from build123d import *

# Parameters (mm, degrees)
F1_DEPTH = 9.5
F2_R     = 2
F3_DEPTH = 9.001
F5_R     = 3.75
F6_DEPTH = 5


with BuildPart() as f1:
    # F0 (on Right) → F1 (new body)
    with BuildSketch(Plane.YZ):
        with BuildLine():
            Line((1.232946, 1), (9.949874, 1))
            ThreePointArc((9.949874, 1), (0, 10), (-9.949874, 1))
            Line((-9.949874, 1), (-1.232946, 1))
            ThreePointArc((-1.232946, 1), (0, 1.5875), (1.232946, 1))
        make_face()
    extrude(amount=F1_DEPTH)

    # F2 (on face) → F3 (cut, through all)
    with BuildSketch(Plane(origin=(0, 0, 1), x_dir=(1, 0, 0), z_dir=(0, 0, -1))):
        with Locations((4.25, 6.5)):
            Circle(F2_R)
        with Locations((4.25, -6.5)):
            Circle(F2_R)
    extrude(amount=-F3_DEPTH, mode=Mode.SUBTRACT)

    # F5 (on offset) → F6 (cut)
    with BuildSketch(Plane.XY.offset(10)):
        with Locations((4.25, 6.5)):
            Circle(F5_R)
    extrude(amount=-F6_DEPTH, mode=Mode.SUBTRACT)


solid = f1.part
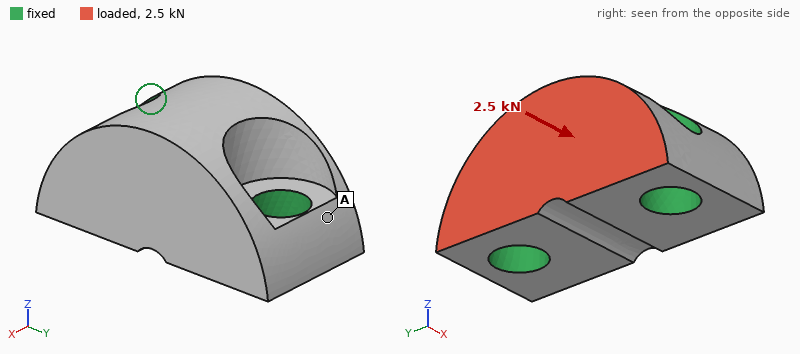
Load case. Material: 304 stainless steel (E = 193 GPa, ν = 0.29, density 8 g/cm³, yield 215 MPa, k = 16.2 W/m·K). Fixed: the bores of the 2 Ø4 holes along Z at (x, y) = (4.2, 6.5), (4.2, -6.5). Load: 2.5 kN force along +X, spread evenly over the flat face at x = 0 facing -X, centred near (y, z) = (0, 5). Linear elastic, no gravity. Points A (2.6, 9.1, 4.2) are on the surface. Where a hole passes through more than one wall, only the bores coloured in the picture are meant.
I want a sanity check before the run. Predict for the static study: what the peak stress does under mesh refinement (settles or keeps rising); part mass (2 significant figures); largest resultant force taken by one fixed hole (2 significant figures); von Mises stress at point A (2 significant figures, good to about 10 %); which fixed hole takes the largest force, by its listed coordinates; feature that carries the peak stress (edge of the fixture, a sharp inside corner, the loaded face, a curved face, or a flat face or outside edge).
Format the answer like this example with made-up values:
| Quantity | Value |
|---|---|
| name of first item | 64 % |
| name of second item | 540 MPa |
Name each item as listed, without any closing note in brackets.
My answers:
| Quantity | Value |
|---|---|
| what the peak stress does under mesh refinement | keeps rising |
| part mass | 8.5 g |
| largest resultant force taken by one fixed hole | 1.4 kN |
| von Mises stress at point A | 28 MPa |
| which fixed hole takes the largest force, by its listed coordinates | (4.2, -6.5) |
| feature that carries the peak stress | a sharp inside corner |
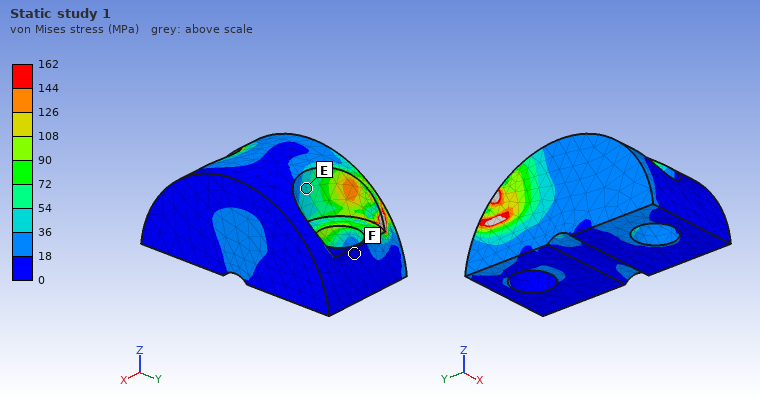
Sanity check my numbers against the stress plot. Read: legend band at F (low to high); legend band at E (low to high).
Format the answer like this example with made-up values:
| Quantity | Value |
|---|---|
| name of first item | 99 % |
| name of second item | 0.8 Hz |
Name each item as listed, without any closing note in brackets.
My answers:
| Quantity | Value |
|---|---|
| legend band at F | 0 to 18 MPa |
| legend band at E | 36 to 54 MPa |
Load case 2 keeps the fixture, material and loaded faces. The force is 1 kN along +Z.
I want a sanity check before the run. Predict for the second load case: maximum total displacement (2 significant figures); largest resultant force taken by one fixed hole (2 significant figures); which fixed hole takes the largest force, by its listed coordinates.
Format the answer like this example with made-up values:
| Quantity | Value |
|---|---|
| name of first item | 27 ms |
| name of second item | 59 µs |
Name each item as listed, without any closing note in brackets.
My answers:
| Quantity | Value |
|---|---|
| maximum total displacement | 2.4 µm |
| largest resultant force taken by one fixed hole | 550 N |
| which fixed hole takes the largest force, by its listed coordinates | (4.2, -6.5) |
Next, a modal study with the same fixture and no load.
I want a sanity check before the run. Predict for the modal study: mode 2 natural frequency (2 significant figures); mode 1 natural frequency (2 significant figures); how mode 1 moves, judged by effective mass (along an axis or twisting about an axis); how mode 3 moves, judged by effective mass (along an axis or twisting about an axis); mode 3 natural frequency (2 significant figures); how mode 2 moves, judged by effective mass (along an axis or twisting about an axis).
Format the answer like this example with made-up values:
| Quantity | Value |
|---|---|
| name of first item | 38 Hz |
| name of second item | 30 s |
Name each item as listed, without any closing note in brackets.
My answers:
| Quantity | Value |
|---|---|
| mode 2 natural frequency | 91 kHz |
| mode 1 natural frequency | 69 kHz |
| how mode 1 moves, judged by effective mass | along X |
| how mode 3 moves, judged by effective mass | along X |
| mode 3 natural frequency | 110 kHz |
| how mode 2 moves, judged by effective mass | along Z |
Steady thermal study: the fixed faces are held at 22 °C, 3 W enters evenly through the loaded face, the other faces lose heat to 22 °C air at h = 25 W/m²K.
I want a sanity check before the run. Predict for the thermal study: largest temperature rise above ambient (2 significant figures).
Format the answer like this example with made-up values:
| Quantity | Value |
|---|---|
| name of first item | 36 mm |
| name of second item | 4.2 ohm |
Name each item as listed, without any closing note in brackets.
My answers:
| Quantity | Value |
|---|---|
| largest temperature rise above ambient | 13 K |
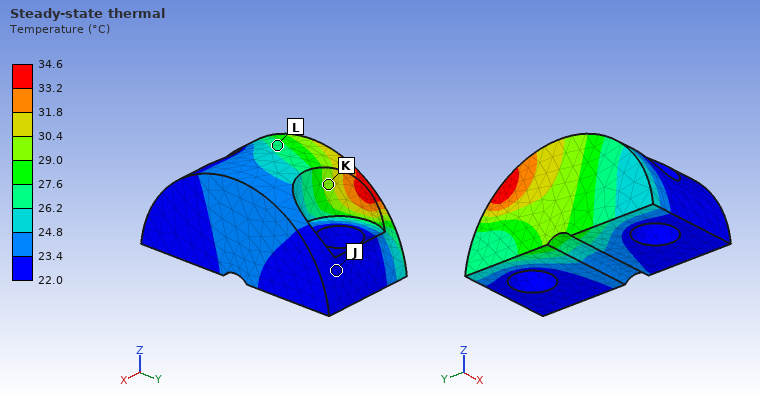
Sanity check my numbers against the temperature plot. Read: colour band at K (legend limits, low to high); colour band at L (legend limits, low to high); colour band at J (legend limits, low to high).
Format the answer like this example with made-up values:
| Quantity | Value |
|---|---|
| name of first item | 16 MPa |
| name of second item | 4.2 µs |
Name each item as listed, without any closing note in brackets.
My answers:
| Quantity | Value |
|---|---|
| colour band at K | 29.0 to 30.4 °C |
| colour band at L | 26.2 to 27.6 °C |
| colour band at J | 22.0 to 23.4 °C |
